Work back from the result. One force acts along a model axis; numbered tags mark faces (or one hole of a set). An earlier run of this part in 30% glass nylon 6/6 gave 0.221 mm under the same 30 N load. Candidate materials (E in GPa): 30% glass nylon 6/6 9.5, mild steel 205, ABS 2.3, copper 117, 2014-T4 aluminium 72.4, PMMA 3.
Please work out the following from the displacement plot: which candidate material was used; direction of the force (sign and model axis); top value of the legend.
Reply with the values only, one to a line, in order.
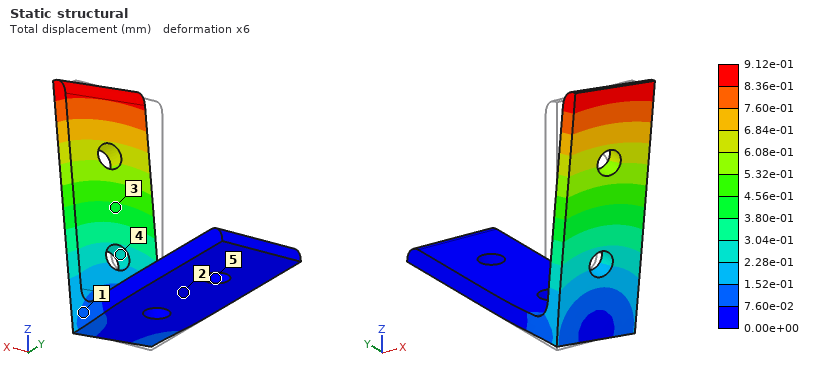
ABS
+X
9.12e-01 mm
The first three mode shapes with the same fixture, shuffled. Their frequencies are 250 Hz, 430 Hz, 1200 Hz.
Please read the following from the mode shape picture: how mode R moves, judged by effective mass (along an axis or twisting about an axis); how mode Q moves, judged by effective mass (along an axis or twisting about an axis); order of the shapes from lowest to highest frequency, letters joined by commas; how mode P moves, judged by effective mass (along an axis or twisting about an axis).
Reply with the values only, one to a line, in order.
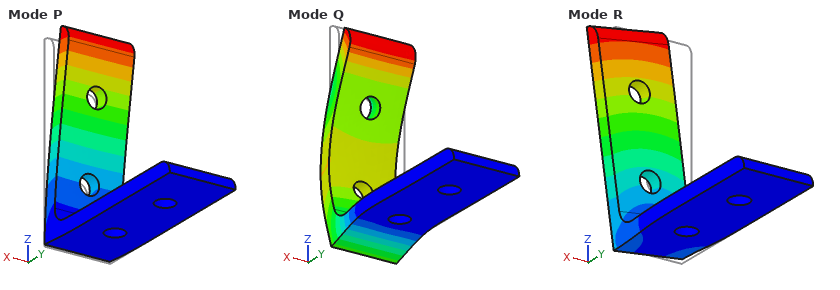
along X
along Z
P, R, Q
along Y
